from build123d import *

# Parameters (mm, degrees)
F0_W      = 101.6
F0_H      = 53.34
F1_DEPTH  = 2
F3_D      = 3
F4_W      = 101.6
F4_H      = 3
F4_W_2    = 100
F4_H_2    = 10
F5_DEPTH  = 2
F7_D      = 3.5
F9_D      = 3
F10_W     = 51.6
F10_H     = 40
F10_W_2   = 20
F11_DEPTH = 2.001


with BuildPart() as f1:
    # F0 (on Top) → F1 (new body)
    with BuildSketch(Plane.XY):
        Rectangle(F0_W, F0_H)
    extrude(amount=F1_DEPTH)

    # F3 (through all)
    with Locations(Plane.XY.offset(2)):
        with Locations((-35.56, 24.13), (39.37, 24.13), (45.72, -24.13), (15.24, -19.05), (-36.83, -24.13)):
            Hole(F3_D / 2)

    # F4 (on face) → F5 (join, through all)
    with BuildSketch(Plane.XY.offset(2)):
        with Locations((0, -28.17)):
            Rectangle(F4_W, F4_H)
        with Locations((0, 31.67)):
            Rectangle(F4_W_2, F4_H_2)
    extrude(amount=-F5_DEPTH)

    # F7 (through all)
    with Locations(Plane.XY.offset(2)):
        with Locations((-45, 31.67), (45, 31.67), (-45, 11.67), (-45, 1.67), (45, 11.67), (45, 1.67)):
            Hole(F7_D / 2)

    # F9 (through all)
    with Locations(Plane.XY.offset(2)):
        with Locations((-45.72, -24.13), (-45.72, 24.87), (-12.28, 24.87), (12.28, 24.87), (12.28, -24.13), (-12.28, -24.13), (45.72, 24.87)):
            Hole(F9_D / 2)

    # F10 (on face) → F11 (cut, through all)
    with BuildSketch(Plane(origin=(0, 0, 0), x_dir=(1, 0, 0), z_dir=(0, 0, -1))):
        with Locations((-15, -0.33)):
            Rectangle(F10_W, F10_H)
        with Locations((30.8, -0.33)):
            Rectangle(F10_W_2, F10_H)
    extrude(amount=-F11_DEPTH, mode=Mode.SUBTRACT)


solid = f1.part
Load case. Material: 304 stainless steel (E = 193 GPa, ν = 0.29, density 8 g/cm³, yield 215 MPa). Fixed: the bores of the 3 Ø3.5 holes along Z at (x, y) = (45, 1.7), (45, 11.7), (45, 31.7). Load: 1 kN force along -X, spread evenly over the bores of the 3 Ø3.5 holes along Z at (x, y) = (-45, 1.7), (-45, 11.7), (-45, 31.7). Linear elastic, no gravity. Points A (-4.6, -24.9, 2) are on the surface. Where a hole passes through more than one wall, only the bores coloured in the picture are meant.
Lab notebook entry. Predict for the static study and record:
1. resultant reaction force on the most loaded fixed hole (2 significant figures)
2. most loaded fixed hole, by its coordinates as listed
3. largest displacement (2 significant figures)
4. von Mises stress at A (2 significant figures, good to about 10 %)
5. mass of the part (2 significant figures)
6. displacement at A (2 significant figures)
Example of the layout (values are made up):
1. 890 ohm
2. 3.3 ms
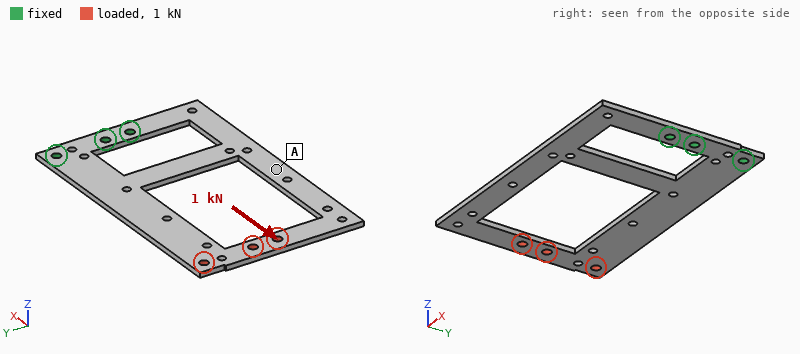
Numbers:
1. 480 N
2. (45, 31.7)
3. 78 µm
4. 13 MPa
5. 59 g
6. 47 µm
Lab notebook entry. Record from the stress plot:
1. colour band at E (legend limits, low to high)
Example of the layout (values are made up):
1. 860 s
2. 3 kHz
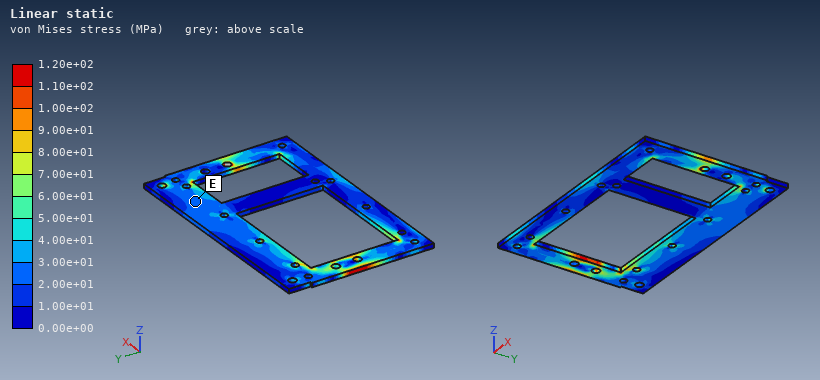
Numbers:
1. 2.00e+01 to 3.00e+01 MPa
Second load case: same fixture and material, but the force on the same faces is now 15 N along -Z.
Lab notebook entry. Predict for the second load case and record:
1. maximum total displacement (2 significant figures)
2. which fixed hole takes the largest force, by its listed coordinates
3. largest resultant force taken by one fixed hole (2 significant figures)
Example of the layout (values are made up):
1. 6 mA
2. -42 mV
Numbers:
1. 1.4 mm
2. (45, 31.7)
3. 16 N
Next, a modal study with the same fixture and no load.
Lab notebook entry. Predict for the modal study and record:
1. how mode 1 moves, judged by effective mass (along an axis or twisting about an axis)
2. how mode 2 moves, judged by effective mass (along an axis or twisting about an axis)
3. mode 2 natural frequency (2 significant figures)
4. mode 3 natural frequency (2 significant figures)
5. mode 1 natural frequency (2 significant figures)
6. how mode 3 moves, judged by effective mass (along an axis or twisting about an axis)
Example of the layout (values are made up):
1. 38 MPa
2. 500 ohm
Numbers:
1. along Z
2. twisting about X
3. 380 Hz
4. 740 Hz
5. 130 Hz
6. along Z
